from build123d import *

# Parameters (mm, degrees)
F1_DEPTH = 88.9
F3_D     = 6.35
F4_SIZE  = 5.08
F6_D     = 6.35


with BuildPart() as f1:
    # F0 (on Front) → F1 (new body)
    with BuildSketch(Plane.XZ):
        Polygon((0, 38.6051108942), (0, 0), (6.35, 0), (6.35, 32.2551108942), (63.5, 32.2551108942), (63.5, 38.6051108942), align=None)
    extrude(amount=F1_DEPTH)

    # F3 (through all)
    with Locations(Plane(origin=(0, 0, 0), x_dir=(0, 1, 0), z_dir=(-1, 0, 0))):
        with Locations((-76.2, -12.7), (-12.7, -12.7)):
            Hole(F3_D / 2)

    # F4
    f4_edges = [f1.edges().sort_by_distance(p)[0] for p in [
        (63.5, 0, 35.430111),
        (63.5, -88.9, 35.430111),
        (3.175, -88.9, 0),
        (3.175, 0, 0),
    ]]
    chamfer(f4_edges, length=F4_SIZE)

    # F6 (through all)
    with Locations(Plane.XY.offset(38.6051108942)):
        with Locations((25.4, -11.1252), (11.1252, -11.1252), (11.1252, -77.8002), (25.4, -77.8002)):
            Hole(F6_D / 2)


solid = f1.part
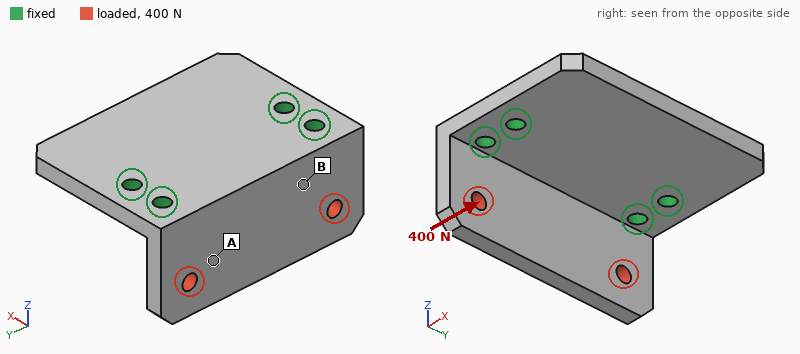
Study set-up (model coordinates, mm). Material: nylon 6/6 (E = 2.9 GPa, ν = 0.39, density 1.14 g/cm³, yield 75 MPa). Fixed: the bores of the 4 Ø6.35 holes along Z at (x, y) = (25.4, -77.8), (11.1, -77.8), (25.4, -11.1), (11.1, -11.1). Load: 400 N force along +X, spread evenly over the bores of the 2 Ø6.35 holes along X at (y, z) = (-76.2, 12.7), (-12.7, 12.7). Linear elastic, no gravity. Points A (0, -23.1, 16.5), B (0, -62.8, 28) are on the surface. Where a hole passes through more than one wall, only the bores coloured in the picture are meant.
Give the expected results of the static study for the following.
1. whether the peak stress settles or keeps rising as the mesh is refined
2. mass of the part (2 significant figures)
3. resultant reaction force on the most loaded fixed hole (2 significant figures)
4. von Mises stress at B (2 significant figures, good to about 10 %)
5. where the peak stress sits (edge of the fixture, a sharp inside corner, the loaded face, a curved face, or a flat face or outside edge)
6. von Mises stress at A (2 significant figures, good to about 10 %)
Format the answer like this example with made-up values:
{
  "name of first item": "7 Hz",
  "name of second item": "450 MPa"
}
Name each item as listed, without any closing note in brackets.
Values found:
{
  "whether the peak stress settles or keeps rising as the mesh is refined": "keeps rising",
  "mass of the part": "60 g",
  "resultant reaction force on the most loaded fixed hole": "190 N",
  "von Mises stress at B": "8.3 MPa",
  "where the peak stress sits": "edge of the fixture",
  "von Mises stress at A": "3.5 MPa"
}
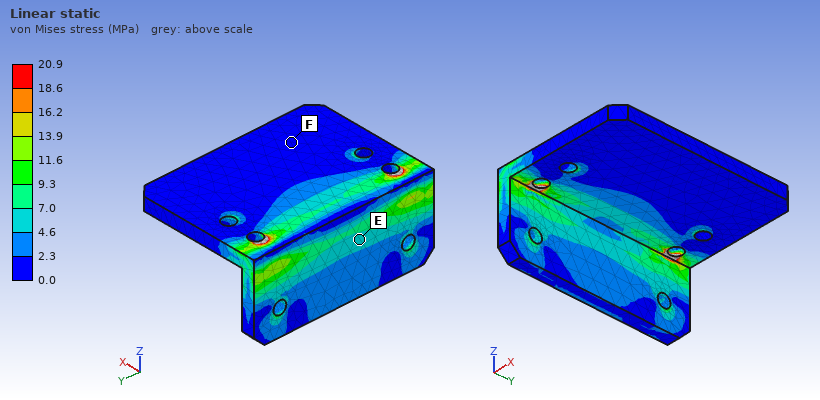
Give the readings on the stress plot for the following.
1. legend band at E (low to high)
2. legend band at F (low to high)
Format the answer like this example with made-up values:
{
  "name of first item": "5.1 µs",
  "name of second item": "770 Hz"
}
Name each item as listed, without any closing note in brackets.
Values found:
{
  "legend band at E": "4.6 to 7.0 MPa",
  "legend band at F": "0.0 to 2.3 MPa"
}
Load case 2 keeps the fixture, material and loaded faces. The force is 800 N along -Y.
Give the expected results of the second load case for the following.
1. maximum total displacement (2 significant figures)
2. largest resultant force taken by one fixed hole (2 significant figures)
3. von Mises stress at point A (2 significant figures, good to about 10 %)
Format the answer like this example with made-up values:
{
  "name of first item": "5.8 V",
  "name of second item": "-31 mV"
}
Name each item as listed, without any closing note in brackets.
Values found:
{
  "maximum total displacement": "0.14 mm",
  "largest resultant force taken by one fixed hole": "430 N",
  "von Mises stress at point A": "2.5 MPa"
}
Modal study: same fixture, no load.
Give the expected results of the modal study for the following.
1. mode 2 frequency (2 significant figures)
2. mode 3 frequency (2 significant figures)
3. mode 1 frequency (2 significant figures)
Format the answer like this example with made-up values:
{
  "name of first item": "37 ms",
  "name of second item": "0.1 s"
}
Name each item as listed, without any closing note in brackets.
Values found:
{
  "mode 2 frequency": "1000 Hz",
  "mode 3 frequency": "1500 Hz",
  "mode 1 frequency": "950 Hz"
}
